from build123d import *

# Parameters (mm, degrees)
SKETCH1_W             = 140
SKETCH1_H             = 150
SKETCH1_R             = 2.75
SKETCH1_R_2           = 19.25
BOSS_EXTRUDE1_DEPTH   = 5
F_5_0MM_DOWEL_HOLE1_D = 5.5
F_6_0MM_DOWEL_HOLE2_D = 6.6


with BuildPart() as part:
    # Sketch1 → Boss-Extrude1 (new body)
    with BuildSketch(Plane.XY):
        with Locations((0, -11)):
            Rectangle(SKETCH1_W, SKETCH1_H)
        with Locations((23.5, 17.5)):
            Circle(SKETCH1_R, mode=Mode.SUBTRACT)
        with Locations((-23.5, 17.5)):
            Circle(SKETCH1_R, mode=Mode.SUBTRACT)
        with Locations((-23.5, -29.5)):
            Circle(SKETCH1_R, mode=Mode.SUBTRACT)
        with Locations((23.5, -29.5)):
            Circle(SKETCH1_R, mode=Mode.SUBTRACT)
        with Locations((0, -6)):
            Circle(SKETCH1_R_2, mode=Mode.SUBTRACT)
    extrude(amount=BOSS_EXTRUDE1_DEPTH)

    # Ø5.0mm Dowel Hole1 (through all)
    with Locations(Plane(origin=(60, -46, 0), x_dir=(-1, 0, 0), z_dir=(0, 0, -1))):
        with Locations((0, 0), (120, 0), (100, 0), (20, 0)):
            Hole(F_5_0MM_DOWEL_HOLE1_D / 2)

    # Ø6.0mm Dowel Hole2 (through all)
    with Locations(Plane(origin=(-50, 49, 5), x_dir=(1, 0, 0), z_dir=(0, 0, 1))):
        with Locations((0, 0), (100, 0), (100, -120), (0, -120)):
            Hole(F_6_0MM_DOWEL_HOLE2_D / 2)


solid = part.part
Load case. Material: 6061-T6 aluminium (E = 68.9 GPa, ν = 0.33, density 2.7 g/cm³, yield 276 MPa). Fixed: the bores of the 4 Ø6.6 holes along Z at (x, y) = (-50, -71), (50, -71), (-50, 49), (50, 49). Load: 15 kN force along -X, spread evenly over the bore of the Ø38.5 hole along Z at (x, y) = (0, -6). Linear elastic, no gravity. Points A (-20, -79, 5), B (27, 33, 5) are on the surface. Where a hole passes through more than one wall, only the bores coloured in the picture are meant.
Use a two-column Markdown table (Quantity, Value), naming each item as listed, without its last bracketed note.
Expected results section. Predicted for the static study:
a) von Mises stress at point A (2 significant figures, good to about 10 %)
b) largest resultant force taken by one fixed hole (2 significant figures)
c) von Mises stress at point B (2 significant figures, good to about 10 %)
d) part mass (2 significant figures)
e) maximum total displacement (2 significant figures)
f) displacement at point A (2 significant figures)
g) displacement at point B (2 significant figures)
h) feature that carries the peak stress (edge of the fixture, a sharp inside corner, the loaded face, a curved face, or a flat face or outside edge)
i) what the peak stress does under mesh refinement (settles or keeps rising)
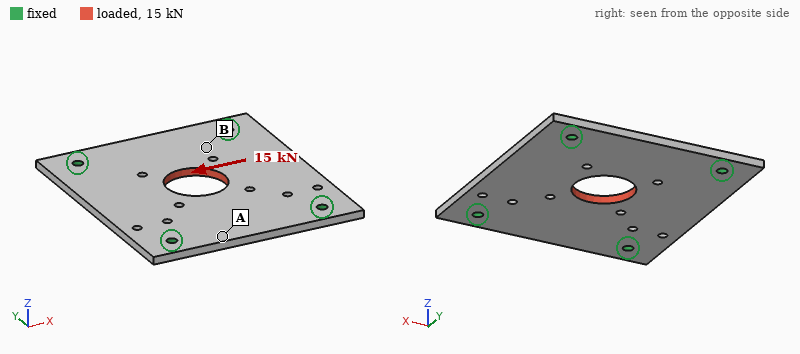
| Quantity | Value |
|---|---|
| von Mises stress at point A | 7.9 MPa |
| largest resultant force taken by one fixed hole | 4.3 kN |
| von Mises stress at point B | 26 MPa |
| part mass | 260 g |
| maximum total displacement | 36 µm |
| displacement at point A | 5.8 µm |
| displacement at point B | 14 µm |
| feature that carries the peak stress | edge of the fixture |
| what the peak stress does under mesh refinement | keeps rising |
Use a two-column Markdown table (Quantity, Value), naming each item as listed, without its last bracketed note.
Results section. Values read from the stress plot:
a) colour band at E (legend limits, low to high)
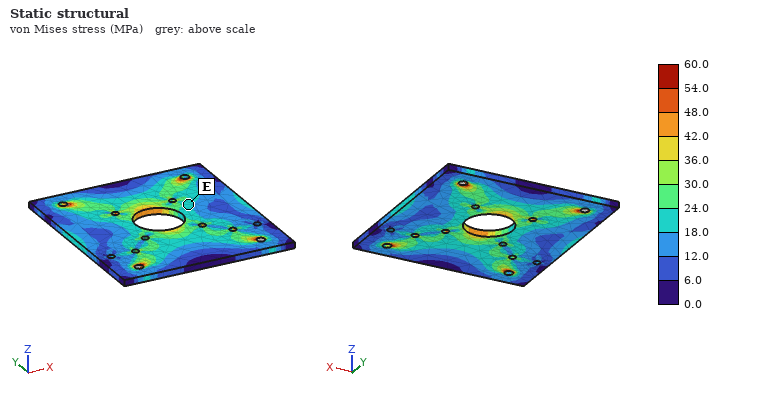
| Quantity | Value |
|---|---|
| colour band at E | 18.0 to 24.0 MPa |
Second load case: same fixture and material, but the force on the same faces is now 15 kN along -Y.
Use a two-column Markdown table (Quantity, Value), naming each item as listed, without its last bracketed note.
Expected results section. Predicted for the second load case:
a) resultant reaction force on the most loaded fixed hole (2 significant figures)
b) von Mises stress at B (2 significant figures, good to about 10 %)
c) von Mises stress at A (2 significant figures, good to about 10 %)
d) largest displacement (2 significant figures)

| Quantity | Value |
|---|---|
| resultant reaction force on the most loaded fixed hole | 4.2 kN |
| von Mises stress at B | 23 MPa |
| von Mises stress at A | 7.4 MPa |
| largest displacement | 30 µm |
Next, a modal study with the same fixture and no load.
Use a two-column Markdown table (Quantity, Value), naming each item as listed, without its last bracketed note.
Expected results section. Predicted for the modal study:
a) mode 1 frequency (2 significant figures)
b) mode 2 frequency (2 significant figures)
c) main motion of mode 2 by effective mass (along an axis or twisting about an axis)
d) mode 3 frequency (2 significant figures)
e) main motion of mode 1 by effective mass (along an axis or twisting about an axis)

| Quantity | Value |
|---|---|
| mode 1 frequency | 1500 Hz |
| mode 2 frequency | 2000 Hz |
| main motion of mode 2 by effective mass | twisting about Y |
| mode 3 frequency | 2300 Hz |
| main motion of mode 1 by effective mass | along Z |
